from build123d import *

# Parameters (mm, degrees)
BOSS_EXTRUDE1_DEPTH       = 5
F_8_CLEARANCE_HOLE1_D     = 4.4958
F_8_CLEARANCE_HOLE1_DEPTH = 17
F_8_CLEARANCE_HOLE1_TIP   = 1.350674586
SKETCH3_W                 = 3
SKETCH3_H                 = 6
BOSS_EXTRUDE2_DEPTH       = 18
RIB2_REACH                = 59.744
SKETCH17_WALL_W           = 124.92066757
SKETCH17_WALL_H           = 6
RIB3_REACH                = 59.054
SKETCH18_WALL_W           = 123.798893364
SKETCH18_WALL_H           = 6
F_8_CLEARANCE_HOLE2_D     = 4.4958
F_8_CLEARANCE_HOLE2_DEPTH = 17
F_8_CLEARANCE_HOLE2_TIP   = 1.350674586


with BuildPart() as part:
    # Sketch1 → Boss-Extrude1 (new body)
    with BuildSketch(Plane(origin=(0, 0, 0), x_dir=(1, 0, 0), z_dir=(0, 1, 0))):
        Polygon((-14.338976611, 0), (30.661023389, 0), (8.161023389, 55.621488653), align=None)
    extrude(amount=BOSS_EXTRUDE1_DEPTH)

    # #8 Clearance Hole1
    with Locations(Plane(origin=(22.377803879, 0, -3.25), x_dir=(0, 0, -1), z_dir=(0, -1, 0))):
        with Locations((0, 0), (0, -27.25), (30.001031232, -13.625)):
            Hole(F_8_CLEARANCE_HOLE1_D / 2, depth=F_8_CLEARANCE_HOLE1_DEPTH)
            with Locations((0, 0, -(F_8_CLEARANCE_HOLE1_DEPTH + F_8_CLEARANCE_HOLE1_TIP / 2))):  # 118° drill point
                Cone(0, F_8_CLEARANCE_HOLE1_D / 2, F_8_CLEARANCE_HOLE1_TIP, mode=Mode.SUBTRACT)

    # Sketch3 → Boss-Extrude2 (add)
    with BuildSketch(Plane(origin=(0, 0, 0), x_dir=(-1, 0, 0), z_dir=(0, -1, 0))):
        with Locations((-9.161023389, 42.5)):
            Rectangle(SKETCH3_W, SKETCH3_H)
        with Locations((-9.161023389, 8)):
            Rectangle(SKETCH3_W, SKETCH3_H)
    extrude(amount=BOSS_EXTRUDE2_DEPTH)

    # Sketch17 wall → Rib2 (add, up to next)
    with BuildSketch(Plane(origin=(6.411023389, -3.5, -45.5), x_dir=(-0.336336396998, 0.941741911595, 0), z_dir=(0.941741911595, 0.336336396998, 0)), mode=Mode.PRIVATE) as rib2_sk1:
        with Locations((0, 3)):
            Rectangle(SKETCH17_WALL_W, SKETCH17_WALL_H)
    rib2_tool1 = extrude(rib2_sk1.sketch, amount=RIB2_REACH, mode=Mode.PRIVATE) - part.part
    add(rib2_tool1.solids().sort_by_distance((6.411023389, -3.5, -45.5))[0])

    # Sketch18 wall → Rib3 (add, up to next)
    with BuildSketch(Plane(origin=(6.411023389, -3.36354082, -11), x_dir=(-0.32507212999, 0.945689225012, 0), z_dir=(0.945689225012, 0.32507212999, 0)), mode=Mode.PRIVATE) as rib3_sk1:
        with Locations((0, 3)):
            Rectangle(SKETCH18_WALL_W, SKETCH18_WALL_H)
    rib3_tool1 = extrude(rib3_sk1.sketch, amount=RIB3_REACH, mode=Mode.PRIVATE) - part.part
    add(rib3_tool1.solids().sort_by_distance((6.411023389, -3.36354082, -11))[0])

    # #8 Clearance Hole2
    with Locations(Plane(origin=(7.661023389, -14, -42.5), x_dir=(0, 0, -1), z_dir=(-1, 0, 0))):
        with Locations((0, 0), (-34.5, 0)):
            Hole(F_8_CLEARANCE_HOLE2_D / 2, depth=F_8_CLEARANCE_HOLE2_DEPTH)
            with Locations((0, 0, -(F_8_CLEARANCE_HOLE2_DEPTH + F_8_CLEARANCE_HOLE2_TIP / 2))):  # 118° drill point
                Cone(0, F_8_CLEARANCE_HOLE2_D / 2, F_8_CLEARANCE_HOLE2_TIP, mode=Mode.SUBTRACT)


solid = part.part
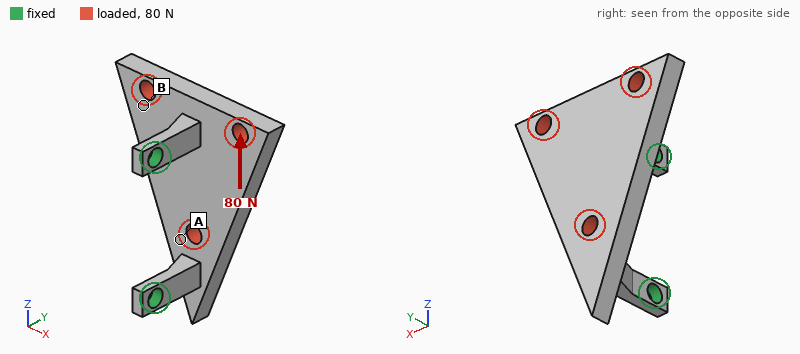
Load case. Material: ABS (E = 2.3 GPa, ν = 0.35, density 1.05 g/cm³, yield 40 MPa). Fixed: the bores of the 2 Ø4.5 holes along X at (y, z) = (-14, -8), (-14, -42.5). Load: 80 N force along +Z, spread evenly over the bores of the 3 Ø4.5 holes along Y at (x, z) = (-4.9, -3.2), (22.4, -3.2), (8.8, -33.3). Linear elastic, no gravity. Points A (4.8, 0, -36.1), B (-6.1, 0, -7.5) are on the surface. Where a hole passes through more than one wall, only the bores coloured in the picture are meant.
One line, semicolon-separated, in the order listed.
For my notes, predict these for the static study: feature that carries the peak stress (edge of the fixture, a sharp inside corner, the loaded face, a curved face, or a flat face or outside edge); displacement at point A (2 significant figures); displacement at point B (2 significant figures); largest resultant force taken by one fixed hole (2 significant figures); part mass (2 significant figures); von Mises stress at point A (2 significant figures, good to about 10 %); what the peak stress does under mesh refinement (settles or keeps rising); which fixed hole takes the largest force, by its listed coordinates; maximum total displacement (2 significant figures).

edge of the fixture; 0.13 mm; 0.12 mm; 47 N; 7.0 g; 3.6 MPa; keeps rising; (-14, -8); 0.16 mm
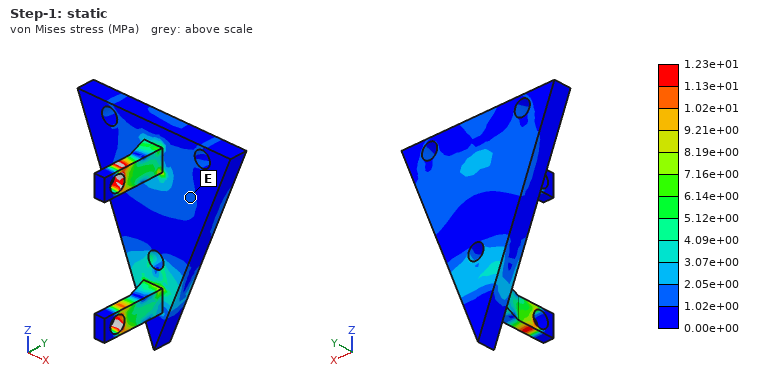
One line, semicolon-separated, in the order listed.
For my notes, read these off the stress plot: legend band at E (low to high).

1.02e+00 to 2.05e+00 MPa
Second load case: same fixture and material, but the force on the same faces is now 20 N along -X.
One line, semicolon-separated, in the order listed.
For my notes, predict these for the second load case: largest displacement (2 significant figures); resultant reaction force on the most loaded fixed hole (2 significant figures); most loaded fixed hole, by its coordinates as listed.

0.81 mm; 16 N; (-14, -8)
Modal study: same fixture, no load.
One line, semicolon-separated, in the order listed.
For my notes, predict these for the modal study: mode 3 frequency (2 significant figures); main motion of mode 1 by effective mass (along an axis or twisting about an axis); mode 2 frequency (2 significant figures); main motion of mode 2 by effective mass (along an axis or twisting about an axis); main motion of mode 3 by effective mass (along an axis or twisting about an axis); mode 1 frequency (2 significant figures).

1500 Hz; along X; 1300 Hz; twisting about Y; along Z; 380 Hz
